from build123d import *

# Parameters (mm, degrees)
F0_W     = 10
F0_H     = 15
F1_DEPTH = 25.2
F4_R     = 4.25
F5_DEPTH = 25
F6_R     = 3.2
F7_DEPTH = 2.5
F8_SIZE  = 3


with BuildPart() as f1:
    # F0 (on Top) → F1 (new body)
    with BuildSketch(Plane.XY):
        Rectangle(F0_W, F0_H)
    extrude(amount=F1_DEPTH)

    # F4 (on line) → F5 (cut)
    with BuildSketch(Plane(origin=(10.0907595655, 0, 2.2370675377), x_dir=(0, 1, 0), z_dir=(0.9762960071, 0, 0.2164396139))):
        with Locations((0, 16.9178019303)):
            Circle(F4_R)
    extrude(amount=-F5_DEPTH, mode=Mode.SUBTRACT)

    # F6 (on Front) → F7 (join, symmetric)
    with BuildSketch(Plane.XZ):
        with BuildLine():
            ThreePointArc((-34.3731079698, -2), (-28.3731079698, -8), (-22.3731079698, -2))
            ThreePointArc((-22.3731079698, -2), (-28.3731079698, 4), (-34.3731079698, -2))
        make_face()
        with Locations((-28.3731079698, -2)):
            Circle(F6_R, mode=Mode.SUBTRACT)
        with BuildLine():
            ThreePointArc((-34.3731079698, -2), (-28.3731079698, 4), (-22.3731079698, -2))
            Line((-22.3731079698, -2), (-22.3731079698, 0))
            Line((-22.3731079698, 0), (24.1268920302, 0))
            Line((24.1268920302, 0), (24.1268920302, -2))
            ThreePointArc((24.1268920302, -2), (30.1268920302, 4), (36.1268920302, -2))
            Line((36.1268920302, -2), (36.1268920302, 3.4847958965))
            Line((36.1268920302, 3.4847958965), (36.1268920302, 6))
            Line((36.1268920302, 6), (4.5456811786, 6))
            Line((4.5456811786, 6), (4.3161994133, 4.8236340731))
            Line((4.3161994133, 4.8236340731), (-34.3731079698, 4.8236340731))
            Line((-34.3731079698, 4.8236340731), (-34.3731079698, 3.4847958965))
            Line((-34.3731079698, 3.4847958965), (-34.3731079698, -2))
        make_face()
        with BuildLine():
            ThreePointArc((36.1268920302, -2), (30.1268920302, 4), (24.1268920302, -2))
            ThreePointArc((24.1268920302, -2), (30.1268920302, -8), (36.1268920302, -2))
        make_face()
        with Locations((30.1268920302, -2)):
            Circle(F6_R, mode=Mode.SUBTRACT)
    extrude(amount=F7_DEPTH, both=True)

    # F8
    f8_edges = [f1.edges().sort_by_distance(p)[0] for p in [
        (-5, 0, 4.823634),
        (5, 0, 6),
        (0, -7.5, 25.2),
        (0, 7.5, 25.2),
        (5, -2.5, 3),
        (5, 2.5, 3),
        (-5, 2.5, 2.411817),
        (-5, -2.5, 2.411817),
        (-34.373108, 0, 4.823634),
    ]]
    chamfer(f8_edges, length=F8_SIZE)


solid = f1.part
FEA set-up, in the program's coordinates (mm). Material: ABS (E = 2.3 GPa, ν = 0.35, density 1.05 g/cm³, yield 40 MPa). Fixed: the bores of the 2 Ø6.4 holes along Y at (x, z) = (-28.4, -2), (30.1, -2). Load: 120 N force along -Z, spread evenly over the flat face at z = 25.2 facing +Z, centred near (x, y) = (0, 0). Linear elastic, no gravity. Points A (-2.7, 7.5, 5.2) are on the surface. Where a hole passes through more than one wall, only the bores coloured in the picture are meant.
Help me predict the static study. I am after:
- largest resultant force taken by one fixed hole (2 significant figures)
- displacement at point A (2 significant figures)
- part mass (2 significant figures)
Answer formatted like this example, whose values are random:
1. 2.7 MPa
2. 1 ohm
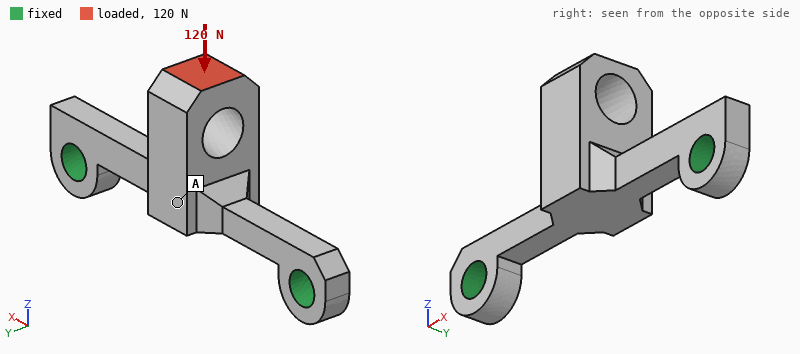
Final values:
1. 80 N
2. 0.35 mm
3. 5.7 g
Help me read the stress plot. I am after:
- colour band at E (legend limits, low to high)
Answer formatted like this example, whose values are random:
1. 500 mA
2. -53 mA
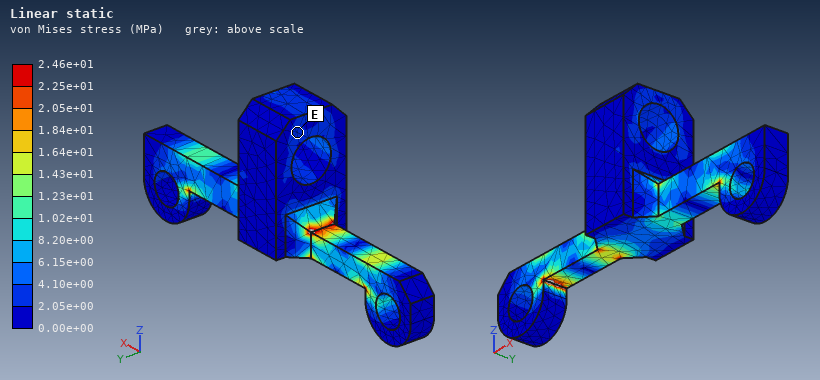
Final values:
1. 2.05e+00 to 4.10e+00 MPa
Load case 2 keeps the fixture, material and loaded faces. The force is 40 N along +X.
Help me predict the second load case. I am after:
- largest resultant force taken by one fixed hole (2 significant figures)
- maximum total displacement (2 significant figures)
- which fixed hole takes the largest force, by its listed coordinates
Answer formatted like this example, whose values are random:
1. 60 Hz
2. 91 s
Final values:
1. 35 N
2. 0.26 mm
3. (30.1, -2)
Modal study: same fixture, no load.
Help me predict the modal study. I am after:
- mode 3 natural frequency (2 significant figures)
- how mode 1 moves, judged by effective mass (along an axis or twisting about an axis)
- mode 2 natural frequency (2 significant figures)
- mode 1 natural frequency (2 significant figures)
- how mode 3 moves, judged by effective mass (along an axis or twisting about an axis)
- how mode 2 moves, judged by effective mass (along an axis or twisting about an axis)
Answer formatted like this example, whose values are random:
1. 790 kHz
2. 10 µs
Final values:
1. 1900 Hz
2. along Y
3. 1500 Hz
4. 630 Hz
5. along Y
6. along Z
